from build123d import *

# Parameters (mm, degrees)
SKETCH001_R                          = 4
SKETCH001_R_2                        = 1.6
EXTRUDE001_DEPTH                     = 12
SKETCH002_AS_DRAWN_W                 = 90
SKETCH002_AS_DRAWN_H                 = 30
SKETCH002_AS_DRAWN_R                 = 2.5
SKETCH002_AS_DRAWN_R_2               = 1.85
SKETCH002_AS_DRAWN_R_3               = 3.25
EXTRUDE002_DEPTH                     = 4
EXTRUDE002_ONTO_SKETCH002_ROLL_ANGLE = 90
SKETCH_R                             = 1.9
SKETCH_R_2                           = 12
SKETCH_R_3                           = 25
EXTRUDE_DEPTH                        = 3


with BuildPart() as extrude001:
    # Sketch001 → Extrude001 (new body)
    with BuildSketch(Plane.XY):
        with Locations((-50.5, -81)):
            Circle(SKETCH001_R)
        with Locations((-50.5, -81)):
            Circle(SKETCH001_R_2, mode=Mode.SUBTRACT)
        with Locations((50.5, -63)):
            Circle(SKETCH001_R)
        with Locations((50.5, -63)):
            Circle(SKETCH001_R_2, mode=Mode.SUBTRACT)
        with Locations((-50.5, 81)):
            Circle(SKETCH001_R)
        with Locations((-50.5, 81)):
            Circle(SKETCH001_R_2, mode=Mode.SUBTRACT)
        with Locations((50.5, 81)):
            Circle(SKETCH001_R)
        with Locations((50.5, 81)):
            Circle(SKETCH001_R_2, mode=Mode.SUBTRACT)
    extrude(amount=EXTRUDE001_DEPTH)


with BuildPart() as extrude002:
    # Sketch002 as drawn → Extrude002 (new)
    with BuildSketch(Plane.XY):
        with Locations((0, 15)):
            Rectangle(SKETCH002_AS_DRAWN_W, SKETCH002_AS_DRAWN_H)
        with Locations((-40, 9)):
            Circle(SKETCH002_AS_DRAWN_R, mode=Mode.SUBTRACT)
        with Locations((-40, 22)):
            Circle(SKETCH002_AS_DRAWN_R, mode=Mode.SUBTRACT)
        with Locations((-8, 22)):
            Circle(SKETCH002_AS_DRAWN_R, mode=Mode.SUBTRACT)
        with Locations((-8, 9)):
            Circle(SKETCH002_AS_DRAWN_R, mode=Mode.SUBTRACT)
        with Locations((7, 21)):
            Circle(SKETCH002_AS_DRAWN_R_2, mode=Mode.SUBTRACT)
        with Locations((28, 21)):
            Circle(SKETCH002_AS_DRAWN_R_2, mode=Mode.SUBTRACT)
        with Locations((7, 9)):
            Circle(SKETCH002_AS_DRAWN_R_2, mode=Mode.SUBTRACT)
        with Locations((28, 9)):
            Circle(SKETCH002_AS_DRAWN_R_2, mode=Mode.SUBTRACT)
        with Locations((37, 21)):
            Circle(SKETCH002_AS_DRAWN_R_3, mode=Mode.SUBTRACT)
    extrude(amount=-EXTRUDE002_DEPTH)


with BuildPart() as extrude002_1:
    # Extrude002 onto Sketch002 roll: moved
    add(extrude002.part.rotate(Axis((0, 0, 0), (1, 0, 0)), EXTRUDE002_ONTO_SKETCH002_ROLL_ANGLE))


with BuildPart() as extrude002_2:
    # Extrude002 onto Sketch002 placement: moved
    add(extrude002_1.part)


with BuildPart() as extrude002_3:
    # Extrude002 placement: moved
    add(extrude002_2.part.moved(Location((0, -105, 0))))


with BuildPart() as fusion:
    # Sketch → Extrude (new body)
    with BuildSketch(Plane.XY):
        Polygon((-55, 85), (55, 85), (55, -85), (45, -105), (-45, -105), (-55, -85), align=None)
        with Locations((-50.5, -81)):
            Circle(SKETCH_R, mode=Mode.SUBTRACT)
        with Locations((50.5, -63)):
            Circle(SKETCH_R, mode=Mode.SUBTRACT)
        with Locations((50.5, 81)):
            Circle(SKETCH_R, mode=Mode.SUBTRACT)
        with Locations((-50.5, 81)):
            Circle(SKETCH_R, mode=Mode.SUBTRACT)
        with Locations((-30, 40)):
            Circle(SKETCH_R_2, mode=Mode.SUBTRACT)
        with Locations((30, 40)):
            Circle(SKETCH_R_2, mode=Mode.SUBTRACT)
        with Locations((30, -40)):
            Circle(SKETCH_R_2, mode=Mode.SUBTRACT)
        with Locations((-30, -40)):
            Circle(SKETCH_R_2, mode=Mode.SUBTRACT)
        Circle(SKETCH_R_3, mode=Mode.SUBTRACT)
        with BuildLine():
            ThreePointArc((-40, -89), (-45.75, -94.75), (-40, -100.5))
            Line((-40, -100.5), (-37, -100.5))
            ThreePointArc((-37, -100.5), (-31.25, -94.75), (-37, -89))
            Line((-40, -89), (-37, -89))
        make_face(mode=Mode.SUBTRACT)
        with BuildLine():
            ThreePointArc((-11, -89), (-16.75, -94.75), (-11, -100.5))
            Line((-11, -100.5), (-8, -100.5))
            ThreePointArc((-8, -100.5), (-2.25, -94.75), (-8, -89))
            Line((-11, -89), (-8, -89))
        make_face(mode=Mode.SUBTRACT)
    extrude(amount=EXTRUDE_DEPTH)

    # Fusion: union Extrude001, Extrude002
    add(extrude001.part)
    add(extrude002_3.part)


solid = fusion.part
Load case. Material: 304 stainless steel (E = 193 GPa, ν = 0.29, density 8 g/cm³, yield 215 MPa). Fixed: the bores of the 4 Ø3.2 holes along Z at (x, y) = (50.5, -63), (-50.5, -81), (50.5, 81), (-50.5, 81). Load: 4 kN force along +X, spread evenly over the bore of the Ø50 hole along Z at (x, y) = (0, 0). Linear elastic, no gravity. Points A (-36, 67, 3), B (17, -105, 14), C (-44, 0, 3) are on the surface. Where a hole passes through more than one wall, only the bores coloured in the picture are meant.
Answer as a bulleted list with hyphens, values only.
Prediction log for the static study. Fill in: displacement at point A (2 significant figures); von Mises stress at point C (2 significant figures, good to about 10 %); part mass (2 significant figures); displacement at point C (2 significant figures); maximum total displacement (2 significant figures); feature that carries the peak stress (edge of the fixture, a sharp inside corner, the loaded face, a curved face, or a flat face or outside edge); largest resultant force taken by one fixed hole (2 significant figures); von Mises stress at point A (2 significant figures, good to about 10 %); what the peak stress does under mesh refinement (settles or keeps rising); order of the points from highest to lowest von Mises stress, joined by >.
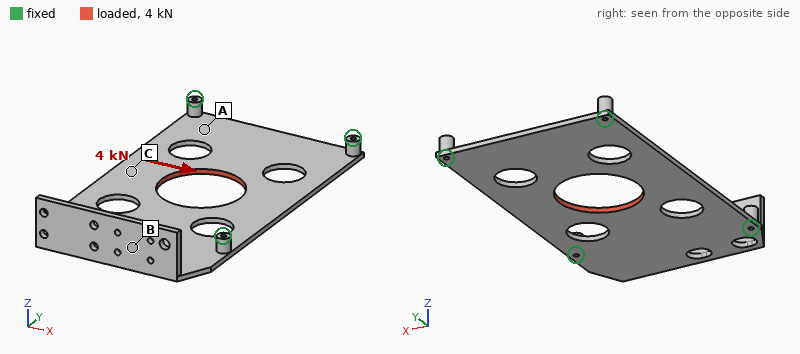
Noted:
- 3.0 µm
- 7.4 MPa
- 480 g
- 13 µm
- 13 µm
- edge of the fixture
- 1.3 kN
- 18 MPa
- keeps rising
- A > C > B
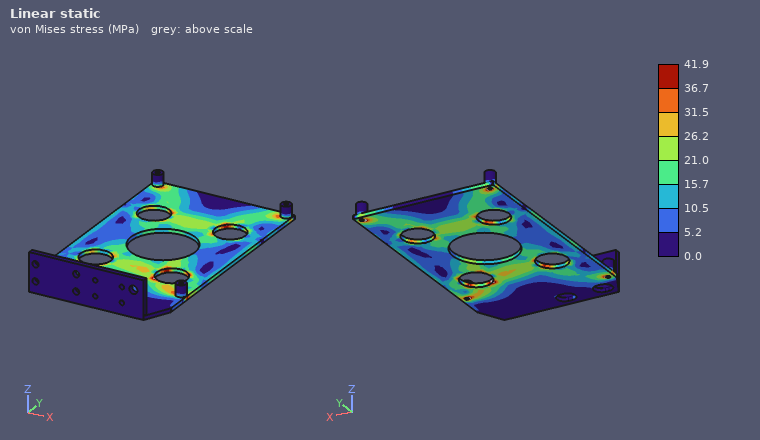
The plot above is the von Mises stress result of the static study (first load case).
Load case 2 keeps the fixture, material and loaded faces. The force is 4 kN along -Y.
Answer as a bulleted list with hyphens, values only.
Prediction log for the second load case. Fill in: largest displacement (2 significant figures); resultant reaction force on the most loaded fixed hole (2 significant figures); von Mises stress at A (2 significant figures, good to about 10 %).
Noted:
- 7.4 µm
- 1.2 kN
- 12 MPa
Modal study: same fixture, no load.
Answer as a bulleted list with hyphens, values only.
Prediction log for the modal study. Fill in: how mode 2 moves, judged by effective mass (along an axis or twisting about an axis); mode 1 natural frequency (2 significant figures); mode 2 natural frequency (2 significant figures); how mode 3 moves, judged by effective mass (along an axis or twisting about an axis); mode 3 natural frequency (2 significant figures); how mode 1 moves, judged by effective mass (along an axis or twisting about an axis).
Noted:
- along Z
- 510 Hz
- 680 Hz
- twisting about Y
- 840 Hz
- along Z
